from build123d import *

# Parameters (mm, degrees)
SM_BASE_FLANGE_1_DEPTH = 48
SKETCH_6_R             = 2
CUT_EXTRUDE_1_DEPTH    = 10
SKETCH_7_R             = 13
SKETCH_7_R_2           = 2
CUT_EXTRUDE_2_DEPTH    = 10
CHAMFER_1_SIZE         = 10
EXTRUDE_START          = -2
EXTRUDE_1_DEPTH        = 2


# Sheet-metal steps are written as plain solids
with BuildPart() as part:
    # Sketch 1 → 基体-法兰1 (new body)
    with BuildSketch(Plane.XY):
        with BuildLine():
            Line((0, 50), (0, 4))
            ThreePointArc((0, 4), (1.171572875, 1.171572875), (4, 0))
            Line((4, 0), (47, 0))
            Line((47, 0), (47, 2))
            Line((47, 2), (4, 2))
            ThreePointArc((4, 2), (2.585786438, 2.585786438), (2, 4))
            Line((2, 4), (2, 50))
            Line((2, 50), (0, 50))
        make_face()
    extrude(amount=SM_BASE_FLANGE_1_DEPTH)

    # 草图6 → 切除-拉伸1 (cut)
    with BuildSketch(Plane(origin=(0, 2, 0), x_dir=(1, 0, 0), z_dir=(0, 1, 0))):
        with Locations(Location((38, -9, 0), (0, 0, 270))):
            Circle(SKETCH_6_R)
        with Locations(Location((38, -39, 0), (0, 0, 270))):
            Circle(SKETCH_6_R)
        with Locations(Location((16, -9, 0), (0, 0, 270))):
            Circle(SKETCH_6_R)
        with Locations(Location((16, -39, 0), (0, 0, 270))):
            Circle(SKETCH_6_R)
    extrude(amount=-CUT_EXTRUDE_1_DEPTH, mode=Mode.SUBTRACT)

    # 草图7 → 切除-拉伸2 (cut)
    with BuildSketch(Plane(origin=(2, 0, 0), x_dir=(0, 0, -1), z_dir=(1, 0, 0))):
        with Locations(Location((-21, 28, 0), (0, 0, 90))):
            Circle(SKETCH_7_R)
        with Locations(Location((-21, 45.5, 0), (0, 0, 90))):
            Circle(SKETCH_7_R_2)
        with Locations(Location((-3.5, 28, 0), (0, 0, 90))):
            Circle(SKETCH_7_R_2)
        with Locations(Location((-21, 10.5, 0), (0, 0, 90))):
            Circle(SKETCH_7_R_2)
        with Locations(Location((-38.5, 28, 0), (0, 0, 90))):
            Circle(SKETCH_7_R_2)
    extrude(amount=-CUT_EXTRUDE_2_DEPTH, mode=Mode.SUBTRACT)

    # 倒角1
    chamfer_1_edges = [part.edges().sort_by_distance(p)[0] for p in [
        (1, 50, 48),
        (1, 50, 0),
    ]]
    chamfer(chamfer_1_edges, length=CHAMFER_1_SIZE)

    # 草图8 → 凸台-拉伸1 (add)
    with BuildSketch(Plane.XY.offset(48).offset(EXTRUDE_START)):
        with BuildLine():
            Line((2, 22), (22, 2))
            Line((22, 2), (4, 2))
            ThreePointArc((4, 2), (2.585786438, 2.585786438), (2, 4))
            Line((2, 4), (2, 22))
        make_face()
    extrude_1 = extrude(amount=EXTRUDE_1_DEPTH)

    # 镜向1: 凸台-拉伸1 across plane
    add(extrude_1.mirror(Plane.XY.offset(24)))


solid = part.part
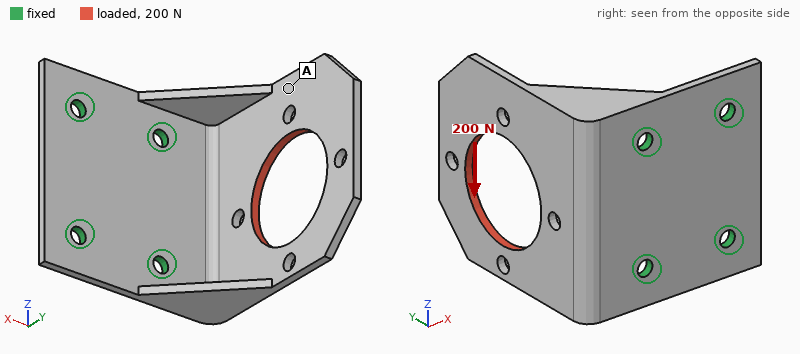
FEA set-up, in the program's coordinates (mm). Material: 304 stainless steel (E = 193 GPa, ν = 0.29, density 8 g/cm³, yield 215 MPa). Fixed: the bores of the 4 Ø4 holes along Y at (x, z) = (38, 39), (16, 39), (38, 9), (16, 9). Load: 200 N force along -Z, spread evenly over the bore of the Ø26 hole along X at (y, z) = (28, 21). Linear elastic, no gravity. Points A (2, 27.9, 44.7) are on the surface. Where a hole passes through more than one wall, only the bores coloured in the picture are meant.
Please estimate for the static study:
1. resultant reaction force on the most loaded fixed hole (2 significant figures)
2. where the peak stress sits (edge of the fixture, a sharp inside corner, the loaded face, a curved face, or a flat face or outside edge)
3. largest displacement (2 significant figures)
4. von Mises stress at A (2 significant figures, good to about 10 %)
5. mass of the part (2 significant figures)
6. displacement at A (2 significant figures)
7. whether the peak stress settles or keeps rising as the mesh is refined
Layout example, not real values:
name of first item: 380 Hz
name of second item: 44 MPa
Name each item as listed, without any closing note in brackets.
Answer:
resultant reaction force on the most loaded fixed hole: 220 N
where the peak stress sits: edge of the fixture
largest displacement: 79 µm
von Mises stress at A: 19 MPa
mass of the part: 67 g
displacement at A: 57 µm
whether the peak stress settles or keeps rising as the mesh is refined: keeps rising
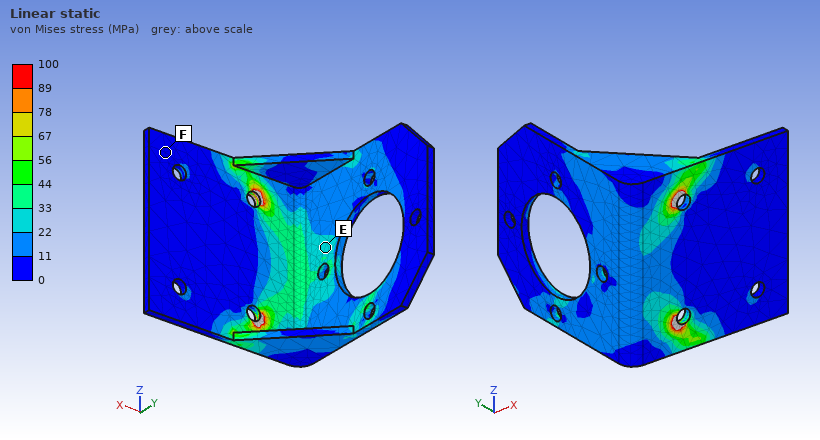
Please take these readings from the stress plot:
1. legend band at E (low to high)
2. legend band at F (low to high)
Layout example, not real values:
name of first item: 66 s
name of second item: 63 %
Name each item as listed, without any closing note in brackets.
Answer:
legend band at E: 22 to 33 MPa
legend band at F: 0 to 11 MPa
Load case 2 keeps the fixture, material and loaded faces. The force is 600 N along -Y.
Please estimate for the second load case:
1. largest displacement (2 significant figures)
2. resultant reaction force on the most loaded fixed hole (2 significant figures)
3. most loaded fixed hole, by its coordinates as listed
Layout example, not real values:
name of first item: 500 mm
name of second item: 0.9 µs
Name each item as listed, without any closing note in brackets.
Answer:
largest displacement: 0.21 mm
resultant reaction force on the most loaded fixed hole: 450 N
most loaded fixed hole, by its coordinates as listed: (16, 9)
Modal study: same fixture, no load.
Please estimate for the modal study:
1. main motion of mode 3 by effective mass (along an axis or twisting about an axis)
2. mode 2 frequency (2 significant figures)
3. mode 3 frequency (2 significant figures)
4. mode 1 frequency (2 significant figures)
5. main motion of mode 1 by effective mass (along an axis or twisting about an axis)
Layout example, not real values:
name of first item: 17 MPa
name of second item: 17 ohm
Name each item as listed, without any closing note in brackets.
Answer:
main motion of mode 3 by effective mass: along Y
mode 2 frequency: 1600 Hz
mode 3 frequency: 2700 Hz
mode 1 frequency: 920 Hz
main motion of mode 1 by effective mass: along X
